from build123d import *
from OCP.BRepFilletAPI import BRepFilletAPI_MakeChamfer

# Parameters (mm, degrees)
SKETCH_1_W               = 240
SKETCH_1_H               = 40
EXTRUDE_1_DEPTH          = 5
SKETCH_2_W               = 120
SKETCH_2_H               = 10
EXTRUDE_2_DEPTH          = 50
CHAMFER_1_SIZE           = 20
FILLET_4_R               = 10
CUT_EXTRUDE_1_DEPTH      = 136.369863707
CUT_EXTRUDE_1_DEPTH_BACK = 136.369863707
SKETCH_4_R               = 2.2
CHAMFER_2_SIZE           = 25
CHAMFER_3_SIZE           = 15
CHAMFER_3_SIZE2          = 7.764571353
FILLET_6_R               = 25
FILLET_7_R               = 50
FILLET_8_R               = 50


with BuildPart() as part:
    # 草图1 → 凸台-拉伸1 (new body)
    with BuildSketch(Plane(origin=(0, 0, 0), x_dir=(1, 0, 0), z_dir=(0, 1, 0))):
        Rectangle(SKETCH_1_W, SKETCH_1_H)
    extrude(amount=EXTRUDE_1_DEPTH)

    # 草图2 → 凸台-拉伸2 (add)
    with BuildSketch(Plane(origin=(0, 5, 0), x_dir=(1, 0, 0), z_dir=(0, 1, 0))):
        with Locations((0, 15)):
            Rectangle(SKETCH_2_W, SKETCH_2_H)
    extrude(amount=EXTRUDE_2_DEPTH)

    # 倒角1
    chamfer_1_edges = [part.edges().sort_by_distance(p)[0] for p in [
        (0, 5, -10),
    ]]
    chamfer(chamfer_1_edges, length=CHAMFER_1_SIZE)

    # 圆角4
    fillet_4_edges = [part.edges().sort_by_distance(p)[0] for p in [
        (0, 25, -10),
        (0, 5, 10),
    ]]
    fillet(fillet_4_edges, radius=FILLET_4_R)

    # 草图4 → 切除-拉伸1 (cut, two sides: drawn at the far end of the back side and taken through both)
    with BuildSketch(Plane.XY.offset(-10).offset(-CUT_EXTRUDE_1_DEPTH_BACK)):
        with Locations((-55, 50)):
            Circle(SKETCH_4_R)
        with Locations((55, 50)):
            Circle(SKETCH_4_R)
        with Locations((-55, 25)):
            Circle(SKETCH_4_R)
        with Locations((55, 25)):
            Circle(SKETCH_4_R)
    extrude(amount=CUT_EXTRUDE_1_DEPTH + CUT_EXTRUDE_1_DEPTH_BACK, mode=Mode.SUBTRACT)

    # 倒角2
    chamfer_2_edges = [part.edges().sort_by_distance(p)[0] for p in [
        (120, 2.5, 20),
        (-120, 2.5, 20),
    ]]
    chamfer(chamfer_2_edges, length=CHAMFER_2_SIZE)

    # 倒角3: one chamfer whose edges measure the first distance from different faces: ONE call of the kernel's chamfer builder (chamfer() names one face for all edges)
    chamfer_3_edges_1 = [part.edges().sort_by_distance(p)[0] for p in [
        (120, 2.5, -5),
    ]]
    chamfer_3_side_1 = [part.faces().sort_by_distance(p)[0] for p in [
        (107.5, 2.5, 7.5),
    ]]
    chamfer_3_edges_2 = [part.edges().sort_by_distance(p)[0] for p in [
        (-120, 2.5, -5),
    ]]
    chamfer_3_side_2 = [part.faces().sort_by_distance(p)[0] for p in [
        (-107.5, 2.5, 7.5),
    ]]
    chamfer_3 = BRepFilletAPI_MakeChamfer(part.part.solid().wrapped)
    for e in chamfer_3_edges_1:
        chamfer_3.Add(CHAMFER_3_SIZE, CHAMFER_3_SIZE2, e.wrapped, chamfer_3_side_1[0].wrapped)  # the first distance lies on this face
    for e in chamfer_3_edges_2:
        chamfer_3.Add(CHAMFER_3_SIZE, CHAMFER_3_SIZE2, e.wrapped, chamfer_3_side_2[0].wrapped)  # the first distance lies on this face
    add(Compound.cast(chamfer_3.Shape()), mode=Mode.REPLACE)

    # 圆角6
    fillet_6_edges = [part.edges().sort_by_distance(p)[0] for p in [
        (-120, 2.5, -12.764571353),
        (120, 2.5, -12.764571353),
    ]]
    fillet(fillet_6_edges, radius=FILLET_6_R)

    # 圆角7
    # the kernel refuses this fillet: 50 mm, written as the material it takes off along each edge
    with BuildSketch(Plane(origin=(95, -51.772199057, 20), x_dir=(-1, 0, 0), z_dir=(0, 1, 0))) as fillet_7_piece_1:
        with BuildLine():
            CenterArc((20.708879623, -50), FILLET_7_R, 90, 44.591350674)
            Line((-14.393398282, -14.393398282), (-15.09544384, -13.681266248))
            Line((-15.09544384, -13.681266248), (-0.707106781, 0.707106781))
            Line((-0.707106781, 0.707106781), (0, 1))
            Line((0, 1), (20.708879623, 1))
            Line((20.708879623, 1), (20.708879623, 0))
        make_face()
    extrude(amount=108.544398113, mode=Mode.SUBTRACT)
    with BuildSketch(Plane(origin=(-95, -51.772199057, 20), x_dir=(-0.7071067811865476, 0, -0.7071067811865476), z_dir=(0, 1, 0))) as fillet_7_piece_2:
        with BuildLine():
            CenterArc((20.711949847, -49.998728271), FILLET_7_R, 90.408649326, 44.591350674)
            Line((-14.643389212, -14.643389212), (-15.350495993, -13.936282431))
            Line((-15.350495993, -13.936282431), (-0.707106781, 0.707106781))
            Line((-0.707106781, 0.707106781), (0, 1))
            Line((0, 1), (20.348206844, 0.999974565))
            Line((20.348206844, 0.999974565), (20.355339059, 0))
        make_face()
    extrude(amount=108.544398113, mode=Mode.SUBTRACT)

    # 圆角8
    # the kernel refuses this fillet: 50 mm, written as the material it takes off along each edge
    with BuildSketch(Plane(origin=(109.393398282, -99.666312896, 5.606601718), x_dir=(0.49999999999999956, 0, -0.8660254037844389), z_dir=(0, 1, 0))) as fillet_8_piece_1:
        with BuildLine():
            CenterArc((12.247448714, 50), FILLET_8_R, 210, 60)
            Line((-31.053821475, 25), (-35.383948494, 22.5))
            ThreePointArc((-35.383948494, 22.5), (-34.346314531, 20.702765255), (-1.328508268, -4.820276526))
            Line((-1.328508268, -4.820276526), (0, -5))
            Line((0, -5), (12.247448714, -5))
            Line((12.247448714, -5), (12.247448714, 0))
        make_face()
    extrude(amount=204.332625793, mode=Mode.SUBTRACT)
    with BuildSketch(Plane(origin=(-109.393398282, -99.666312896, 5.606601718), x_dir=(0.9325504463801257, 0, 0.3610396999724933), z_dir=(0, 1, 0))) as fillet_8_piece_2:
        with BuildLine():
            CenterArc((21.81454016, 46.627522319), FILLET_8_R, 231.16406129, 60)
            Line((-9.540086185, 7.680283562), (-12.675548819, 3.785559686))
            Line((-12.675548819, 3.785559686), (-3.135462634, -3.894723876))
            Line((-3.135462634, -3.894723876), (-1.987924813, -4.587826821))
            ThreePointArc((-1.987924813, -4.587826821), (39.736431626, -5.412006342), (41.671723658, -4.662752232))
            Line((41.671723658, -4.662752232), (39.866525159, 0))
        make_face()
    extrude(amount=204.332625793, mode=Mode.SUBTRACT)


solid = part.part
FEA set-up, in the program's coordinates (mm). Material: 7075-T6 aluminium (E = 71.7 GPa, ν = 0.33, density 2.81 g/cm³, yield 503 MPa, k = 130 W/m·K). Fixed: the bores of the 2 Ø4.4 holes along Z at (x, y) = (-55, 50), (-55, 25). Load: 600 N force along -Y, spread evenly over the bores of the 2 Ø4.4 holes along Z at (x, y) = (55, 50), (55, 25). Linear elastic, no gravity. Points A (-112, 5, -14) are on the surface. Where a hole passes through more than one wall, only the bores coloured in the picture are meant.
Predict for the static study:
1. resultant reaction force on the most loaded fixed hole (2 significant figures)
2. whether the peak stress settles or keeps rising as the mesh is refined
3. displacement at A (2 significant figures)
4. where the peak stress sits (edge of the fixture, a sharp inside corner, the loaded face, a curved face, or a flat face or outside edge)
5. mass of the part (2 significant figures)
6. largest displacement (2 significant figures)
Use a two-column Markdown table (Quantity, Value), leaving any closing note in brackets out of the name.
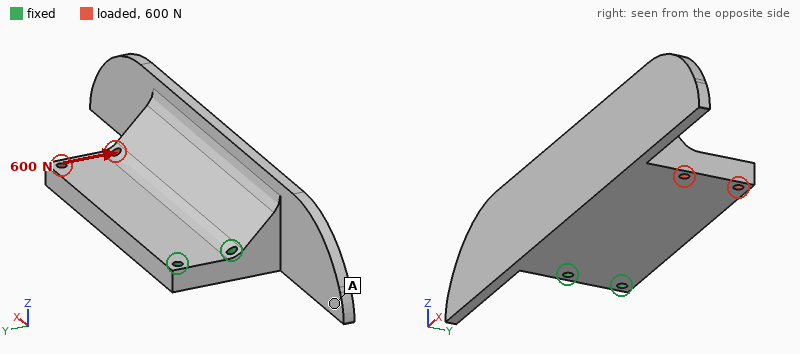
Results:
| Quantity | Value |
|---|---|
| resultant reaction force on the most loaded fixed hole | 2.5 kN |
| whether the peak stress settles or keeps rising as the mesh is refined | keeps rising |
| displacement at A | 0.028 mm |
| where the peak stress sits | edge of the fixture |
| mass of the part | 360 g |
| largest displacement | 0.10 mm |
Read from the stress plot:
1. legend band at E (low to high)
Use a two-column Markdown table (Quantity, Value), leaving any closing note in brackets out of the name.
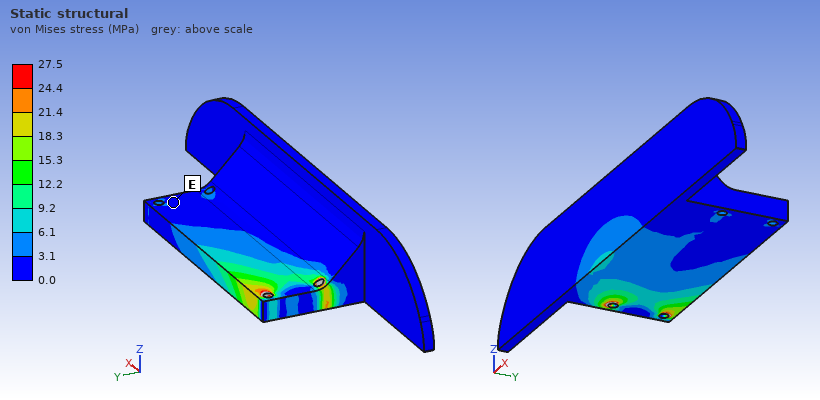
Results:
| Quantity | Value |
|---|---|
| legend band at E | 0.0 to 3.1 MPa |
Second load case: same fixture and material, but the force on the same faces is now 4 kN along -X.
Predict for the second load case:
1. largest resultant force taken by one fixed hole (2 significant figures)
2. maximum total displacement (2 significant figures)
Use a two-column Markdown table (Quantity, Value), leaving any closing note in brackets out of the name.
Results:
| Quantity | Value |
|---|---|
| largest resultant force taken by one fixed hole | 2.1 kN |
| maximum total displacement | 45 µm |
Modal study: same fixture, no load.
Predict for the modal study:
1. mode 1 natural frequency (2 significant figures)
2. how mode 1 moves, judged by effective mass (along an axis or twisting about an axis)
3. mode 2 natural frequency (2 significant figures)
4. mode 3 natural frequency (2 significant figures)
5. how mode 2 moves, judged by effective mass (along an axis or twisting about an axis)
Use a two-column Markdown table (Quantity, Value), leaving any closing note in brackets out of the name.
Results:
| Quantity | Value |
|---|---|
| mode 1 natural frequency | 530 Hz |
| how mode 1 moves, judged by effective mass | along Z |
| mode 2 natural frequency | 1100 Hz |
| mode 3 natural frequency | 1300 Hz |
| how mode 2 moves, judged by effective mass | along Y |
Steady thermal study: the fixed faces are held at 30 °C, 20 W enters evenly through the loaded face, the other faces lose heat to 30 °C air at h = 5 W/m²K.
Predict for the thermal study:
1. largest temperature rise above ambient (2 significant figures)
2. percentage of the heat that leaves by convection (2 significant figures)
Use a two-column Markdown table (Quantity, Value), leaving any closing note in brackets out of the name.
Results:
| Quantity | Value |
|---|---|
| largest temperature rise above ambient | 27 K |
| percentage of the heat that leaves by convection | 8.8 % |
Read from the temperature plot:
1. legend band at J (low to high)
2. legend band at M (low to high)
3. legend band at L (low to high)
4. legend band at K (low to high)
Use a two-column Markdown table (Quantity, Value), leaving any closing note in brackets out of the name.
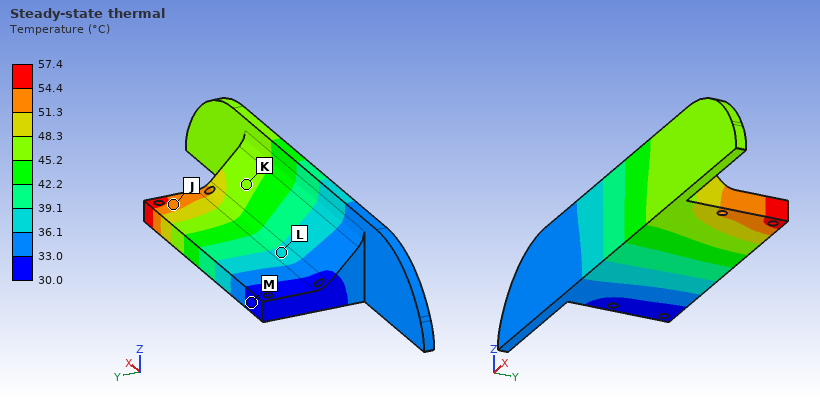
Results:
| Quantity | Value |
|---|---|
| legend band at J | 51.3 to 54.4 °C |
| legend band at M | 30.0 to 33.0 °C |
| legend band at L | 36.1 to 39.1 °C |
| legend band at K | 45.2 to 48.3 °C |
